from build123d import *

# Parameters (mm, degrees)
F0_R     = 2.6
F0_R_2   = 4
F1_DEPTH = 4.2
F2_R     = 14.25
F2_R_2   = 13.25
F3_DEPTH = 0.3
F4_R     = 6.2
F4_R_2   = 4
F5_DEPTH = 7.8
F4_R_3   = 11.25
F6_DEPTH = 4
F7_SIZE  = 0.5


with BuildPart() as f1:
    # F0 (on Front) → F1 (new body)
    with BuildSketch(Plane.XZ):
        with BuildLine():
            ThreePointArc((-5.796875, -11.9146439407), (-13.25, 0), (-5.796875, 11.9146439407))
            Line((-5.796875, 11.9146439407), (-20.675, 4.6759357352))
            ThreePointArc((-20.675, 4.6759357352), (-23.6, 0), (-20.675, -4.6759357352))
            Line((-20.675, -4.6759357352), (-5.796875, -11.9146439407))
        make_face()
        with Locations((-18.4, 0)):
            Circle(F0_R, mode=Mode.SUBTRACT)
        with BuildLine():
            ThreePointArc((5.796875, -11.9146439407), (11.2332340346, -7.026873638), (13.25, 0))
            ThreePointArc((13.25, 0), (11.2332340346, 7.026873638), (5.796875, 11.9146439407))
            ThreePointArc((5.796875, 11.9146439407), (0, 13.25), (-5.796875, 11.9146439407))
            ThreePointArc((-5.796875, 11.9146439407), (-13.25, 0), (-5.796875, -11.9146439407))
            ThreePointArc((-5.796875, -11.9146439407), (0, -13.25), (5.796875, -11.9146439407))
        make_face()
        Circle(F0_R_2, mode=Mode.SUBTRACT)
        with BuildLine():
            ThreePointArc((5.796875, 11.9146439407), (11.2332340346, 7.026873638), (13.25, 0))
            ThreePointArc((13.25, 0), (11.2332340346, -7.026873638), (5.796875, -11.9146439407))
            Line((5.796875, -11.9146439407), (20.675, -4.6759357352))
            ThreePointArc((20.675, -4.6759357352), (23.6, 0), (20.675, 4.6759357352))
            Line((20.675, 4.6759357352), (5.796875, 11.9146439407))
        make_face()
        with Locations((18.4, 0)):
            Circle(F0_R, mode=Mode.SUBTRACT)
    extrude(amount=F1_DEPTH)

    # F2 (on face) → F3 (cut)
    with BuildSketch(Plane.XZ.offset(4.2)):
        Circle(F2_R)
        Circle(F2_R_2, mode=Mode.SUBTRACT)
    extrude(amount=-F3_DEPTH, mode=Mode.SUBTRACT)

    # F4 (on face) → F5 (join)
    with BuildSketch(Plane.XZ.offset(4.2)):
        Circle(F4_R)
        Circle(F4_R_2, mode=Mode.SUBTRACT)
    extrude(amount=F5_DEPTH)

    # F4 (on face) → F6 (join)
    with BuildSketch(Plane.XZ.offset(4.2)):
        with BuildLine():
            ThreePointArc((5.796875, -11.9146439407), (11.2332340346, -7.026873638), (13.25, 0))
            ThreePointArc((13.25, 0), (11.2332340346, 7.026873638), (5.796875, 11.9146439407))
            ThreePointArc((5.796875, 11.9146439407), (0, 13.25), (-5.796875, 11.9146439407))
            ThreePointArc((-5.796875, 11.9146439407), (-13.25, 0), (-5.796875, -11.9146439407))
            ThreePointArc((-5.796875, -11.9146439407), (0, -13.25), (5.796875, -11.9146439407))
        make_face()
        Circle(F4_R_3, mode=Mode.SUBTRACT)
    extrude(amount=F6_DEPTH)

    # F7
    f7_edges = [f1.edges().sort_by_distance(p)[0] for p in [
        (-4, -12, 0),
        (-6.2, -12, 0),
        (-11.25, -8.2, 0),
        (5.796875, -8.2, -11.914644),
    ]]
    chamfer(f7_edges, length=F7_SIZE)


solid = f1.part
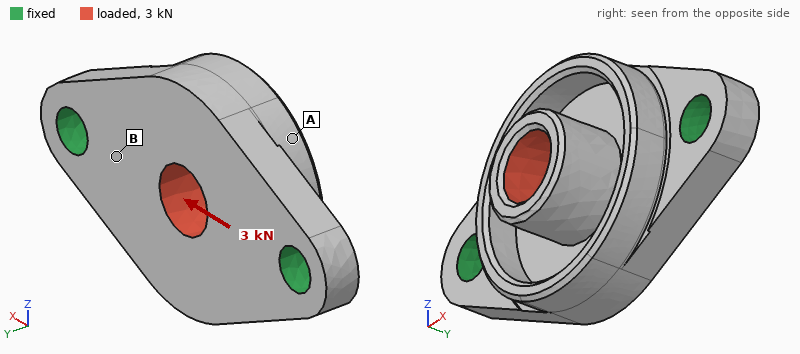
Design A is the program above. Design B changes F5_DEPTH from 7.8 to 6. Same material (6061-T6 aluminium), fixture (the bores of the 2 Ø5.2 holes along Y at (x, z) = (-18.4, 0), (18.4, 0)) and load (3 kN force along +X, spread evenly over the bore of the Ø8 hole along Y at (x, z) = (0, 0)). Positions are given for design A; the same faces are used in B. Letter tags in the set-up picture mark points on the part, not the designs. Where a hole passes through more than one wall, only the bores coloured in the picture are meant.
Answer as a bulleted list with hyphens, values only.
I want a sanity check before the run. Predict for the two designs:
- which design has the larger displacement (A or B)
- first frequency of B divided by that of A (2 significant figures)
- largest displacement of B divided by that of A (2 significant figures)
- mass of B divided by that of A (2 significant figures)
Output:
- A
- 1.0
- 0.69
- 0.97
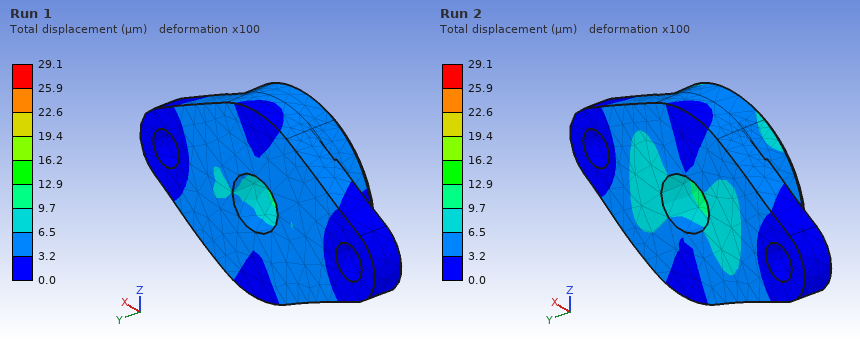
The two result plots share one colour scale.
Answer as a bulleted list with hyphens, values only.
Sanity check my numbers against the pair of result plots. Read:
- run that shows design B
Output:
- Run 1
